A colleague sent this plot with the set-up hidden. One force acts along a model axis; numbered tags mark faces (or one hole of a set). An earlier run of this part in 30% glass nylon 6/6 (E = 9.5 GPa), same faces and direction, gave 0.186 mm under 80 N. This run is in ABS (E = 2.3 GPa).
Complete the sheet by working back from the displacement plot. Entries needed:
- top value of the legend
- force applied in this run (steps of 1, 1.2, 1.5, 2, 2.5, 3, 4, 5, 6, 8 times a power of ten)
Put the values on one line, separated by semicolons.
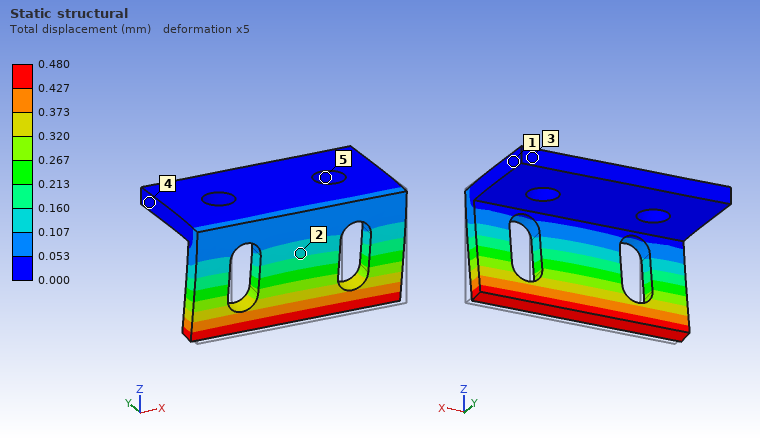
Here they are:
0.480 mm; 50 N
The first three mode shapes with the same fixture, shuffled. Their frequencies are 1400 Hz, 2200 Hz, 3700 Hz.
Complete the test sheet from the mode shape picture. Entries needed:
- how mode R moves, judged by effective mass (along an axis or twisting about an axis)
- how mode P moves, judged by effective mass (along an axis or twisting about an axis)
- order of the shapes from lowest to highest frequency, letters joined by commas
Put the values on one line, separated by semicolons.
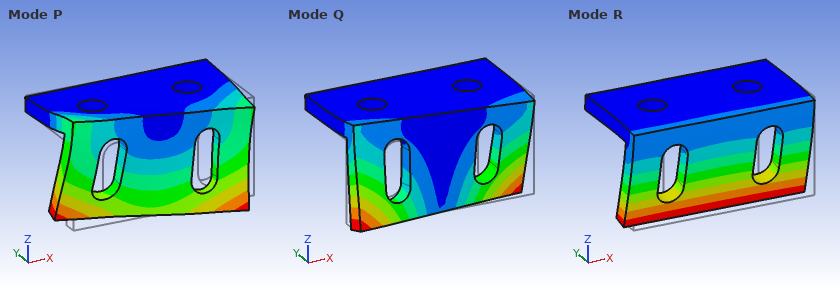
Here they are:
along Y; along X; R, Q, P
